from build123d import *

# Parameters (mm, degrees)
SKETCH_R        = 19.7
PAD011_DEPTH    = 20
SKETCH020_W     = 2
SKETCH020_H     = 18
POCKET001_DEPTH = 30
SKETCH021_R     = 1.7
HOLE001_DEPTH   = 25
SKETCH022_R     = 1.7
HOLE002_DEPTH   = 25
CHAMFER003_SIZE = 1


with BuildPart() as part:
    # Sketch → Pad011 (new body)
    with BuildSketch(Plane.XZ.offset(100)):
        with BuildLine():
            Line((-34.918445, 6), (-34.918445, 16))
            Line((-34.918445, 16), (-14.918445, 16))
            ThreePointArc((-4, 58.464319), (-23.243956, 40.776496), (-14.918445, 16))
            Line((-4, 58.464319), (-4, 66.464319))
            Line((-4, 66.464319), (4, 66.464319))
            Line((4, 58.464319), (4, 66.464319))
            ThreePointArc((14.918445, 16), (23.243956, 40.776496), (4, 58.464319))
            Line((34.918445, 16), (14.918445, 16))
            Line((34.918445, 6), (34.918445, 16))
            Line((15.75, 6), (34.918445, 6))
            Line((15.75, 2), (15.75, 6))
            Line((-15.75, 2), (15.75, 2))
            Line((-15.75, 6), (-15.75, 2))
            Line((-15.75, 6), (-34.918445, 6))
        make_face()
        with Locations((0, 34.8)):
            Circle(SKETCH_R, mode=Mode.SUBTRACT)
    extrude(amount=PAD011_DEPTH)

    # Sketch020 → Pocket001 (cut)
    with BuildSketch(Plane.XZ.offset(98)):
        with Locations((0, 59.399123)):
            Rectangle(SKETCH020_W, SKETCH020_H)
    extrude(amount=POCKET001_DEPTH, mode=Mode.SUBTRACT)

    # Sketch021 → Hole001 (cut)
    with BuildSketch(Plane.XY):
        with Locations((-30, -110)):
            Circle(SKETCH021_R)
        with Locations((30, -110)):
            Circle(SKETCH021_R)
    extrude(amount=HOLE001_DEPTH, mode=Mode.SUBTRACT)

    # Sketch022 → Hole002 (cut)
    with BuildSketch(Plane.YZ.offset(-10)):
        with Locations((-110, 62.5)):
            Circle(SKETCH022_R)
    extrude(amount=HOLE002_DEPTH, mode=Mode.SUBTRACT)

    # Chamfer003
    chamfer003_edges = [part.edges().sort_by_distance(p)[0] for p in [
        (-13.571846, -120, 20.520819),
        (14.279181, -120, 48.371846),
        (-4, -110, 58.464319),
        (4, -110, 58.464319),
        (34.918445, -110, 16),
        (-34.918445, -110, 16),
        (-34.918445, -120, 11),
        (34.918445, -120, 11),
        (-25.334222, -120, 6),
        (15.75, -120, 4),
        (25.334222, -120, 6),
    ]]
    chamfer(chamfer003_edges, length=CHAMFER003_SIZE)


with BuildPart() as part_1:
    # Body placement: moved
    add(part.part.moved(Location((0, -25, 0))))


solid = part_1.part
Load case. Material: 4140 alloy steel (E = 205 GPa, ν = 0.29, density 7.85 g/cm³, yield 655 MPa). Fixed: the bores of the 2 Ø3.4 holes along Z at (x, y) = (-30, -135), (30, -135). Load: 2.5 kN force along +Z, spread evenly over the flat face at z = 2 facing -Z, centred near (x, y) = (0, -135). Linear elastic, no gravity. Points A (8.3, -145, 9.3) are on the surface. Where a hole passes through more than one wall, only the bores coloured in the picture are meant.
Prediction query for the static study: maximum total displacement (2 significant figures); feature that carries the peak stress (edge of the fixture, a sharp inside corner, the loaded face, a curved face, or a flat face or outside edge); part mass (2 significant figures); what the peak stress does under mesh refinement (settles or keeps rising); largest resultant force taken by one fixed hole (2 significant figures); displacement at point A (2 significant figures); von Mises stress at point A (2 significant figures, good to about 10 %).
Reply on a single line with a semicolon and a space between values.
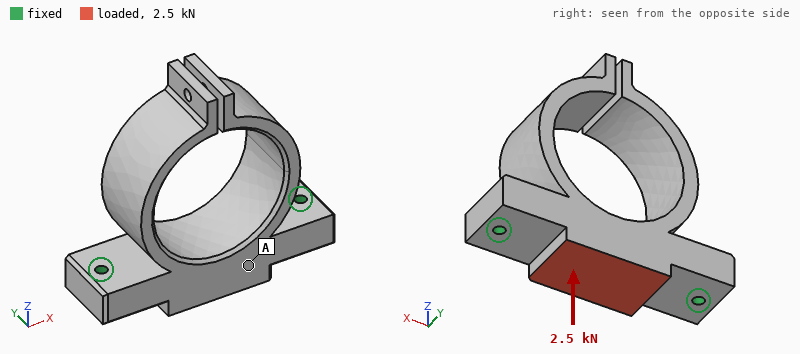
13 µm; edge of the fixture; 210 g; keeps rising; 1.3 kN; 6.3 µm; 8.3 MPa
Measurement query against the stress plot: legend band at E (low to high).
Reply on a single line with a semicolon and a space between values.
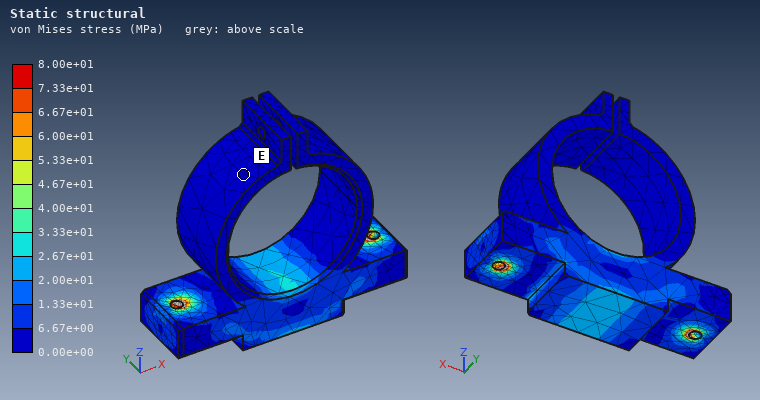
0.00e+00 to 6.67e+00 MPa
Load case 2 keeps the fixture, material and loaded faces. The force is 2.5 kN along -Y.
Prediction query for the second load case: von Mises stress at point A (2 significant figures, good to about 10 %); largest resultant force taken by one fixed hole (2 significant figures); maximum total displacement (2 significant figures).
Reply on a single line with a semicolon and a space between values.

27 MPa; 1.3 kN; 22 µm
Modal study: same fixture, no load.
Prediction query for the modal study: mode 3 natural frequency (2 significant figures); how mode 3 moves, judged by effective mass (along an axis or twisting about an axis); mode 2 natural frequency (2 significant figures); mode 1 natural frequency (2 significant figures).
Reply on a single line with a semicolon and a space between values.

1800 Hz; along Y; 1100 Hz; 1100 Hz
